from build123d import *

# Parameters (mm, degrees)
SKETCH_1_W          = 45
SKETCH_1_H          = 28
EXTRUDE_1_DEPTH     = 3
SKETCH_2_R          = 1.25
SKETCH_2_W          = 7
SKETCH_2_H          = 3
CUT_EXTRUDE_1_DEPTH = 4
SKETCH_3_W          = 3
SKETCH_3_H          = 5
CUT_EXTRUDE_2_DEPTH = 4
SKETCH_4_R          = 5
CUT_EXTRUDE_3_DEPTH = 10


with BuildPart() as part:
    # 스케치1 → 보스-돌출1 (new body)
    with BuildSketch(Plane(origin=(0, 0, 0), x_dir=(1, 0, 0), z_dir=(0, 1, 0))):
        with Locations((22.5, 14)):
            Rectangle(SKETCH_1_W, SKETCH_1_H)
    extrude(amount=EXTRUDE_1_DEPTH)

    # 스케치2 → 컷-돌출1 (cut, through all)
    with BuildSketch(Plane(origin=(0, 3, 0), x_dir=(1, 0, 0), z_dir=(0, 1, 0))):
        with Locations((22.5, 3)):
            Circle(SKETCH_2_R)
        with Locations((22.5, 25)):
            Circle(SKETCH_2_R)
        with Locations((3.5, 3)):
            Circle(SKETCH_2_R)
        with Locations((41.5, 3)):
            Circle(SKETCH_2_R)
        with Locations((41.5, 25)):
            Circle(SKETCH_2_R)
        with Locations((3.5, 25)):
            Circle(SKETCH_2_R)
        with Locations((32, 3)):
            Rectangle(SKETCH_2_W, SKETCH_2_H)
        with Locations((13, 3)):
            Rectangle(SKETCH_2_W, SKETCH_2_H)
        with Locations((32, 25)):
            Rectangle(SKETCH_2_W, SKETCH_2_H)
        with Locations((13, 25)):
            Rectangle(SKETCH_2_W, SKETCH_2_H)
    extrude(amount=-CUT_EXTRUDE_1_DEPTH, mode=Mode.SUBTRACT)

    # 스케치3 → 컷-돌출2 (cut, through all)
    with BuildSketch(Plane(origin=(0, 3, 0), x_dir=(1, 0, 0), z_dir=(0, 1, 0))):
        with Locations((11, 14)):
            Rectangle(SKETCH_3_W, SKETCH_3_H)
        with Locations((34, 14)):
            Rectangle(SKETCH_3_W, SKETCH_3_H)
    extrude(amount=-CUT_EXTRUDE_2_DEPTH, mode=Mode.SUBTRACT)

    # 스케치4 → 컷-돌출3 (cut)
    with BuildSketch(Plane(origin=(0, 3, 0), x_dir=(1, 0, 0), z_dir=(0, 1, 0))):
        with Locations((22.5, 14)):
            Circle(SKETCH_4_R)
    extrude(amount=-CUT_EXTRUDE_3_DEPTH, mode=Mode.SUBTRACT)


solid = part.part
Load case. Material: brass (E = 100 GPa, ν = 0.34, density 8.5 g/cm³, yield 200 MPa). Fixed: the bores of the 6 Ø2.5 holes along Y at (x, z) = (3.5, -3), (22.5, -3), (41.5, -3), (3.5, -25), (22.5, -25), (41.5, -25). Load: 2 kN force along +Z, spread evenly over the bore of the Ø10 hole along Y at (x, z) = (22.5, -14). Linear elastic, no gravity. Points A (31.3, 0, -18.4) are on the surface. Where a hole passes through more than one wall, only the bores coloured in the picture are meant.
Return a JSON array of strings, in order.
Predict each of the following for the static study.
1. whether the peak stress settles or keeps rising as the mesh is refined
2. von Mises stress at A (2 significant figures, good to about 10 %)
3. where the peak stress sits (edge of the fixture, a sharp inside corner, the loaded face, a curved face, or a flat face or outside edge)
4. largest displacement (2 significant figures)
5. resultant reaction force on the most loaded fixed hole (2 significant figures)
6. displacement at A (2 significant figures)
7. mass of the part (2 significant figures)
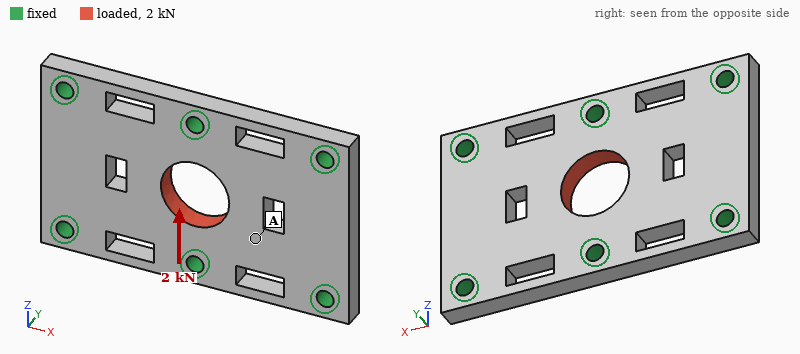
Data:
["keeps rising", "9.0 MPa", "edge of the fixture", "2.9 µm", "780 N", "1.6 µm", "26 g"]
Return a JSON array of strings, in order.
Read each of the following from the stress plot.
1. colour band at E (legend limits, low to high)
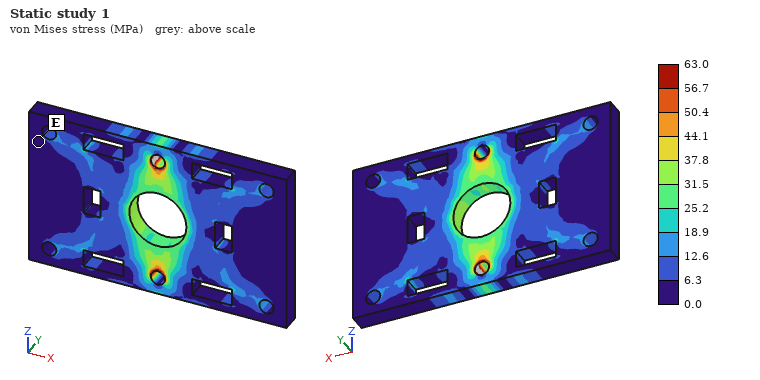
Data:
["0.0 to 6.3 MPa"]
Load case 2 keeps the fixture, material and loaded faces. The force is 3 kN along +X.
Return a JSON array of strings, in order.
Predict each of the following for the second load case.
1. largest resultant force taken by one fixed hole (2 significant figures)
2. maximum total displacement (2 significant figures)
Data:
["760 N", "5.2 µm"]
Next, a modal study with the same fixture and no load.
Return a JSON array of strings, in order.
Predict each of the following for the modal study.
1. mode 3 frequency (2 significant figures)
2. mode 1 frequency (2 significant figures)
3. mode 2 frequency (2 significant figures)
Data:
["24 kHz", "17 kHz", "17 kHz"]
